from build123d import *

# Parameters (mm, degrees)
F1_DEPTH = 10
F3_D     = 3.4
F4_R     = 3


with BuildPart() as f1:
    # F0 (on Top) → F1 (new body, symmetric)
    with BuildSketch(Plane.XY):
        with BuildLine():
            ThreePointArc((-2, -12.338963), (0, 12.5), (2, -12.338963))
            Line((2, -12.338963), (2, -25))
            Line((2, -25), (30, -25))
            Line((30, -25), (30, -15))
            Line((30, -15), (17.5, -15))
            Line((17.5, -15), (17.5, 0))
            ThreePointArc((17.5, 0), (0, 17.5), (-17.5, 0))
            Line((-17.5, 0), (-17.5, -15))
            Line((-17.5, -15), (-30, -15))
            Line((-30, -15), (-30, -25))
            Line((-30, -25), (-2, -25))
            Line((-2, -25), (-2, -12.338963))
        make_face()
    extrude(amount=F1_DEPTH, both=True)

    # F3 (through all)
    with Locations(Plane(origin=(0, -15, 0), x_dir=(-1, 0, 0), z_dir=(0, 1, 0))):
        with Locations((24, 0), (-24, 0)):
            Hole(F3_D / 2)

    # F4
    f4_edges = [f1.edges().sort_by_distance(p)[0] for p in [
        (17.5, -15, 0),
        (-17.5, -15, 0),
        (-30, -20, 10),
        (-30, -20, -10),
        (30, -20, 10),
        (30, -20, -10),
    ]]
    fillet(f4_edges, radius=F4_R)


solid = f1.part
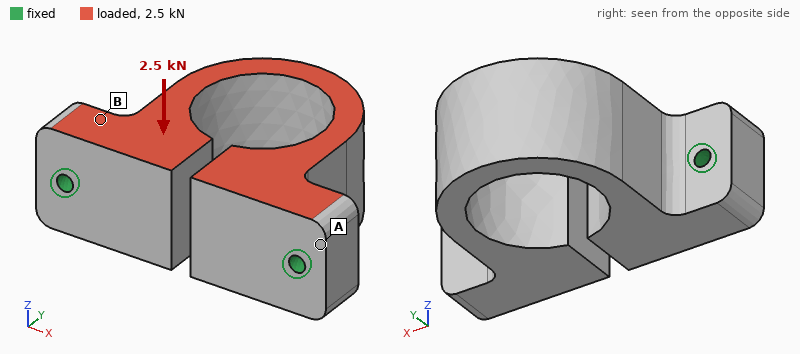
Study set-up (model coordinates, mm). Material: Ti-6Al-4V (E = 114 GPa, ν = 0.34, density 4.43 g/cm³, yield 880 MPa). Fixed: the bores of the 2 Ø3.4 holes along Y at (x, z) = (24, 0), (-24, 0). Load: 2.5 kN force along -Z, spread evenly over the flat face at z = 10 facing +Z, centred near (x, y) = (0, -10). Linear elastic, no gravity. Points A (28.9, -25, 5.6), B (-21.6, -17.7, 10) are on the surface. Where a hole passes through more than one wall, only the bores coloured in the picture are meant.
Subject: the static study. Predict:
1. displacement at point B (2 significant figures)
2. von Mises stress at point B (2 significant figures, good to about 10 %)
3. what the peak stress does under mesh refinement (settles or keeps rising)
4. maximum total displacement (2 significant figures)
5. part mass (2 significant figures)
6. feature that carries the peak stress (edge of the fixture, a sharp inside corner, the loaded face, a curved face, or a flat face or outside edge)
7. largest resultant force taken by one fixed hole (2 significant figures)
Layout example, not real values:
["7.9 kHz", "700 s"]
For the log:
["9.0 µm", "29 MPa", "keeps rising", "44 µm", "94 g", "edge of the fixture", "1.3 kN"]
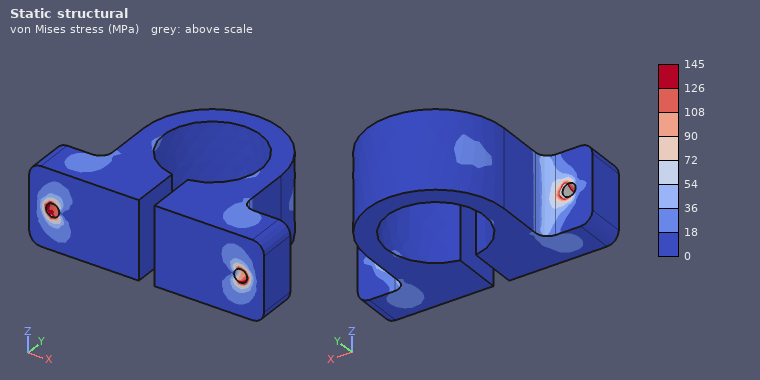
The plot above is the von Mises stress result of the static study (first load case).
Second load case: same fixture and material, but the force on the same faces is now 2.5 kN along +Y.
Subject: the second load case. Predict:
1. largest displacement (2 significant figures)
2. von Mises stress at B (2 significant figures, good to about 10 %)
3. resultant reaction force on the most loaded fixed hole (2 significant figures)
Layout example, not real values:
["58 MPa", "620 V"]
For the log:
["31 µm", "24 MPa", "1.3 kN"]
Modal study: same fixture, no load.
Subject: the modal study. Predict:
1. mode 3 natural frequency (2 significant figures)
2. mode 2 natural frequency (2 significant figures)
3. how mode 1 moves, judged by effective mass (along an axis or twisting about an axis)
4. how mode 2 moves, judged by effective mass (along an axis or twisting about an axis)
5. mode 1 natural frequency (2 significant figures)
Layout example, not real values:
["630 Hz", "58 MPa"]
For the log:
["8800 Hz", "6200 Hz", "along Z", "along X", "5100 Hz"]
